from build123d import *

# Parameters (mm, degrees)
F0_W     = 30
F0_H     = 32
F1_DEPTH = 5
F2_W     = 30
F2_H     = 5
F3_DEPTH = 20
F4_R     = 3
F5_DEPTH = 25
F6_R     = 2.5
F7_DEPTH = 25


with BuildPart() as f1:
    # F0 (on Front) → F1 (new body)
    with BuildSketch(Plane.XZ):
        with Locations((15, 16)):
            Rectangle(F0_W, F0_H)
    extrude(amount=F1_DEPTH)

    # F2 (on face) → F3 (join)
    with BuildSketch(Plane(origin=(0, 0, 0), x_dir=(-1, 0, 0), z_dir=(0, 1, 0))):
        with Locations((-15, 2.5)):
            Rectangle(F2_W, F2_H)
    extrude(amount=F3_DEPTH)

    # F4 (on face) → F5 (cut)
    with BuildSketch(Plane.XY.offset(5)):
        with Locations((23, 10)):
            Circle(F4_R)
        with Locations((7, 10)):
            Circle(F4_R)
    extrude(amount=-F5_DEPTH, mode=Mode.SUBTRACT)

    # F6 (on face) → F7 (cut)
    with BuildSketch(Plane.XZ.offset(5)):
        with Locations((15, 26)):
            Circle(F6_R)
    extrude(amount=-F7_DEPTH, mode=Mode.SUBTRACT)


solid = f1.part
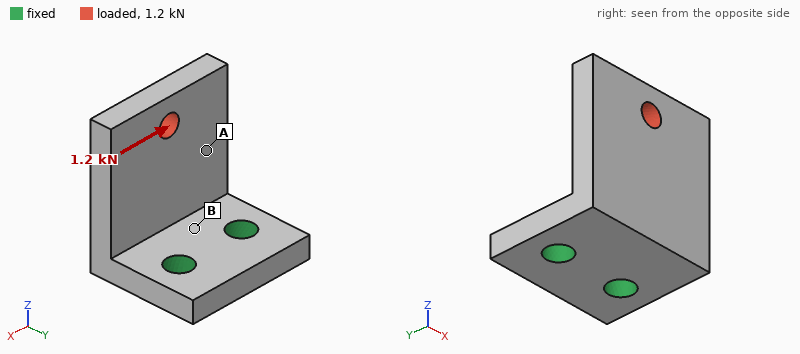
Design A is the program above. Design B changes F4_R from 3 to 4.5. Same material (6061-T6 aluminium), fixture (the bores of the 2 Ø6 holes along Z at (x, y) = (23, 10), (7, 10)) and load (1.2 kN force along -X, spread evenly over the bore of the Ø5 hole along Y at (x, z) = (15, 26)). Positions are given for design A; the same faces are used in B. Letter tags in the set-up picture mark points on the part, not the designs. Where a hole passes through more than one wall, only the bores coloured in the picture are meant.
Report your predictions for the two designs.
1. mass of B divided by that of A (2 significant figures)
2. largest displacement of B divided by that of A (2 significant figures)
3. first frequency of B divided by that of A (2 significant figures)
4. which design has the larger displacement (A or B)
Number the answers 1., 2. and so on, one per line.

1. 0.95
2. 0.76
3. 1.1
4. A
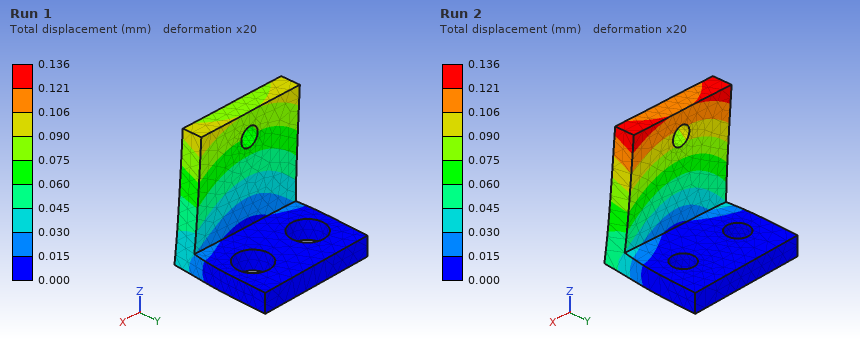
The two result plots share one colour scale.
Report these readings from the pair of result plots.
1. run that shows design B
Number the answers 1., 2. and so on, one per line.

1. Run 1
